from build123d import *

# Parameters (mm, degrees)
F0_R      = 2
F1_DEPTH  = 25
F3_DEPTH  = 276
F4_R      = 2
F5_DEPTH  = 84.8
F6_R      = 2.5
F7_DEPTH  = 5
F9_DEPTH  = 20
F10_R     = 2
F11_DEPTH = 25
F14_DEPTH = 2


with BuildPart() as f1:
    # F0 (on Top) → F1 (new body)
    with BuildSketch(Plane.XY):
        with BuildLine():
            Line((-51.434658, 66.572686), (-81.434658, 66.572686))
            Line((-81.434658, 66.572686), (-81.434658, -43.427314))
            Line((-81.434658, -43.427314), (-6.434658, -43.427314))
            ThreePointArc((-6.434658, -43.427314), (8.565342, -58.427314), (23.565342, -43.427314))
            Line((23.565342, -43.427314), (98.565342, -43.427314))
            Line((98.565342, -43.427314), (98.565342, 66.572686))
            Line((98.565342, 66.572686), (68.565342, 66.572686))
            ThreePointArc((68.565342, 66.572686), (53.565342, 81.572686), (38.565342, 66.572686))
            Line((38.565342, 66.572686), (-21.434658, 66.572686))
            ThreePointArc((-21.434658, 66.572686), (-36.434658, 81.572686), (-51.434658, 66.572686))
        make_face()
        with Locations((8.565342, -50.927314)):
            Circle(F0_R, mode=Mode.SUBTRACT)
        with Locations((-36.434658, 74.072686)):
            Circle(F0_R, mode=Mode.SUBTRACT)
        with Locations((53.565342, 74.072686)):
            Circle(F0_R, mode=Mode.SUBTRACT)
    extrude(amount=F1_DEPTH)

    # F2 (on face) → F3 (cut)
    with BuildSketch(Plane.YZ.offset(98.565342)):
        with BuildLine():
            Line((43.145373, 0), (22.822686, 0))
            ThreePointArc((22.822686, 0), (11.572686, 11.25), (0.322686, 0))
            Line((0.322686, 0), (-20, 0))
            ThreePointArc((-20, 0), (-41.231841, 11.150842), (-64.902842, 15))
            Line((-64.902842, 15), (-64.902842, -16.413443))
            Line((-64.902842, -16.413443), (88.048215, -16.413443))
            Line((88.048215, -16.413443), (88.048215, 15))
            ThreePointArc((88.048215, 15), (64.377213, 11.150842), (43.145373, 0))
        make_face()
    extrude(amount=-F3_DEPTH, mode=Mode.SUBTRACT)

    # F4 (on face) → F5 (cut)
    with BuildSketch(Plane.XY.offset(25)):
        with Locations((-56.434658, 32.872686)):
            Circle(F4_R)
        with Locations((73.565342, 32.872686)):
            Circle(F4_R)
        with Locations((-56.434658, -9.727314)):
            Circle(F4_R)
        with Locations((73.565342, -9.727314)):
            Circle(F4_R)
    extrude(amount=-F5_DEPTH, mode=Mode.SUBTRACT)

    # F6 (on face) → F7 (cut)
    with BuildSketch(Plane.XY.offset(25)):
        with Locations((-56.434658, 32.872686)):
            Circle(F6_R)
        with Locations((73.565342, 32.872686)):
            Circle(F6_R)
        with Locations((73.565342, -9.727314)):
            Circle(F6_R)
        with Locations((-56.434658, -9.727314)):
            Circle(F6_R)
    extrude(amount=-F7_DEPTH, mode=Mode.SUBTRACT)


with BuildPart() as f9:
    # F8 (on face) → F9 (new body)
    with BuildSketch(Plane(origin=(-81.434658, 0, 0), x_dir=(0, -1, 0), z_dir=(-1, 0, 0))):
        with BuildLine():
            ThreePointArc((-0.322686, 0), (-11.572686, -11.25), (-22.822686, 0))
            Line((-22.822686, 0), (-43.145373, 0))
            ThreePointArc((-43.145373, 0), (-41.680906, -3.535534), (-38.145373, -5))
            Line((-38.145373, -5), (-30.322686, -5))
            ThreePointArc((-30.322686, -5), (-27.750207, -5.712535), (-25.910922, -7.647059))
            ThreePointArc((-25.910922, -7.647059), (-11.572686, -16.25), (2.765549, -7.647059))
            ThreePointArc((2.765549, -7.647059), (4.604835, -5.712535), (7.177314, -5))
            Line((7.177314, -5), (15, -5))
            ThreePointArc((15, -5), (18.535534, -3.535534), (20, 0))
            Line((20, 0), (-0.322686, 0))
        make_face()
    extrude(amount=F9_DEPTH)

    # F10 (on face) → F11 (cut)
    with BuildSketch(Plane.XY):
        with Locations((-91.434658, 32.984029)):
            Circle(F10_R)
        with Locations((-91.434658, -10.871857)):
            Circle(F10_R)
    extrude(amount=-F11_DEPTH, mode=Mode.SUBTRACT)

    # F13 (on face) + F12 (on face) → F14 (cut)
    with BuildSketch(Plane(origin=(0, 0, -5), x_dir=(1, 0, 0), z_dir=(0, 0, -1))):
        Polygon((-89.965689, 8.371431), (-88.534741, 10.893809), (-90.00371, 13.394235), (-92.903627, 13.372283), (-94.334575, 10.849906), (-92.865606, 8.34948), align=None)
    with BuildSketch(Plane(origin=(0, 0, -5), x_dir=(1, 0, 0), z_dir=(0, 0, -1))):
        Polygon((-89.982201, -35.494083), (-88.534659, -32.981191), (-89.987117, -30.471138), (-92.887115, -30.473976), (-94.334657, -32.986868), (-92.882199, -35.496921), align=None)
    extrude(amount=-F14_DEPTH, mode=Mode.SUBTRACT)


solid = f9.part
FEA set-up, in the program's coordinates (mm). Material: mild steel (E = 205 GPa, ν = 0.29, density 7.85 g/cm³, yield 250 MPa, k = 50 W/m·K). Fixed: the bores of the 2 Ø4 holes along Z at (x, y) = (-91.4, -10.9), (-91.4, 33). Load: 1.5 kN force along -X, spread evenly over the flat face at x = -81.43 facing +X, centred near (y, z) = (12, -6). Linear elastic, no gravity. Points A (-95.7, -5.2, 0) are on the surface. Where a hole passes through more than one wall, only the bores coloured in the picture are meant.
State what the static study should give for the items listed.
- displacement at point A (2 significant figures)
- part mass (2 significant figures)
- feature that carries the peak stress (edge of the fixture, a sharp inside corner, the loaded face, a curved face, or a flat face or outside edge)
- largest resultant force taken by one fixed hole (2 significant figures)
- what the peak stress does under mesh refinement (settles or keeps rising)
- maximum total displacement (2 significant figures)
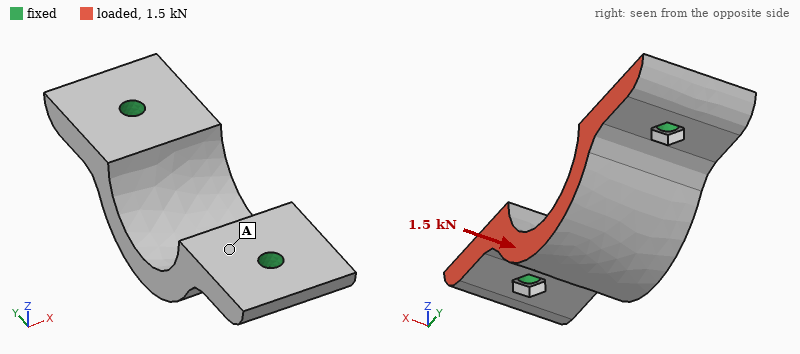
2.7 µm
56 g
edge of the fixture
770 N
keeps rising
17 µm
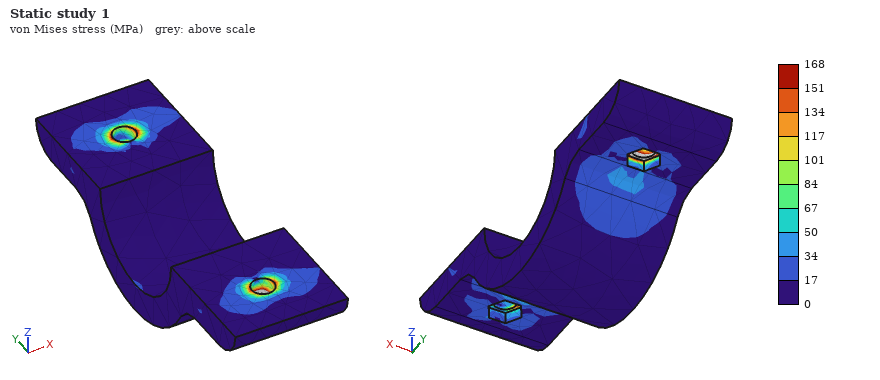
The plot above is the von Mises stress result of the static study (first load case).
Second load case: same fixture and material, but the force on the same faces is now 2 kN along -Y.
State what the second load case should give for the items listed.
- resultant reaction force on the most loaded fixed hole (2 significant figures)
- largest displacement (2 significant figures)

1.1 kN
6.3 µm
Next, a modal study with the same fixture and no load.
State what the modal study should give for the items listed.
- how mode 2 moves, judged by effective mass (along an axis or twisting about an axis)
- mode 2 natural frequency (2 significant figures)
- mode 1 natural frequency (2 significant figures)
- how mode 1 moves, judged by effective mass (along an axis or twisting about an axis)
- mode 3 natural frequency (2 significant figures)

along Z
17 kHz
7200 Hz
along X
19 kHz
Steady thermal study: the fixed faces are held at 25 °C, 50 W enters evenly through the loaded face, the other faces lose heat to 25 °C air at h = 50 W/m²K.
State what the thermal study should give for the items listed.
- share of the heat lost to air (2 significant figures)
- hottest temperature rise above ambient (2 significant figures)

12 %
72 K
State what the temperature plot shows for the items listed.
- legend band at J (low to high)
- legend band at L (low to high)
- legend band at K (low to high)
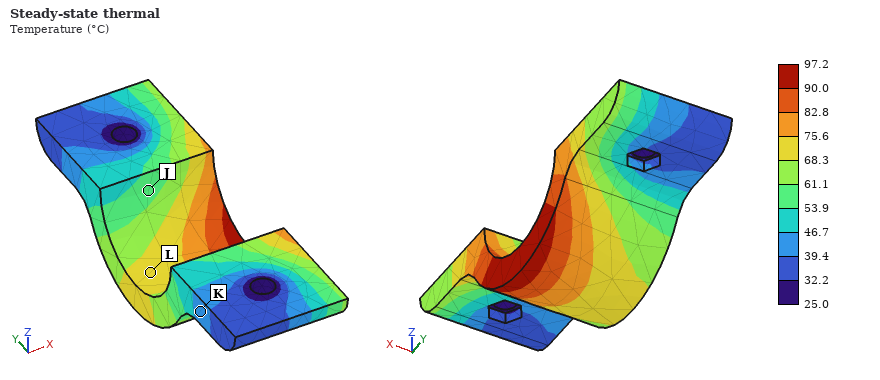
53.9 to 61.1 °C
68.3 to 75.6 °C
39.4 to 46.7 °C
